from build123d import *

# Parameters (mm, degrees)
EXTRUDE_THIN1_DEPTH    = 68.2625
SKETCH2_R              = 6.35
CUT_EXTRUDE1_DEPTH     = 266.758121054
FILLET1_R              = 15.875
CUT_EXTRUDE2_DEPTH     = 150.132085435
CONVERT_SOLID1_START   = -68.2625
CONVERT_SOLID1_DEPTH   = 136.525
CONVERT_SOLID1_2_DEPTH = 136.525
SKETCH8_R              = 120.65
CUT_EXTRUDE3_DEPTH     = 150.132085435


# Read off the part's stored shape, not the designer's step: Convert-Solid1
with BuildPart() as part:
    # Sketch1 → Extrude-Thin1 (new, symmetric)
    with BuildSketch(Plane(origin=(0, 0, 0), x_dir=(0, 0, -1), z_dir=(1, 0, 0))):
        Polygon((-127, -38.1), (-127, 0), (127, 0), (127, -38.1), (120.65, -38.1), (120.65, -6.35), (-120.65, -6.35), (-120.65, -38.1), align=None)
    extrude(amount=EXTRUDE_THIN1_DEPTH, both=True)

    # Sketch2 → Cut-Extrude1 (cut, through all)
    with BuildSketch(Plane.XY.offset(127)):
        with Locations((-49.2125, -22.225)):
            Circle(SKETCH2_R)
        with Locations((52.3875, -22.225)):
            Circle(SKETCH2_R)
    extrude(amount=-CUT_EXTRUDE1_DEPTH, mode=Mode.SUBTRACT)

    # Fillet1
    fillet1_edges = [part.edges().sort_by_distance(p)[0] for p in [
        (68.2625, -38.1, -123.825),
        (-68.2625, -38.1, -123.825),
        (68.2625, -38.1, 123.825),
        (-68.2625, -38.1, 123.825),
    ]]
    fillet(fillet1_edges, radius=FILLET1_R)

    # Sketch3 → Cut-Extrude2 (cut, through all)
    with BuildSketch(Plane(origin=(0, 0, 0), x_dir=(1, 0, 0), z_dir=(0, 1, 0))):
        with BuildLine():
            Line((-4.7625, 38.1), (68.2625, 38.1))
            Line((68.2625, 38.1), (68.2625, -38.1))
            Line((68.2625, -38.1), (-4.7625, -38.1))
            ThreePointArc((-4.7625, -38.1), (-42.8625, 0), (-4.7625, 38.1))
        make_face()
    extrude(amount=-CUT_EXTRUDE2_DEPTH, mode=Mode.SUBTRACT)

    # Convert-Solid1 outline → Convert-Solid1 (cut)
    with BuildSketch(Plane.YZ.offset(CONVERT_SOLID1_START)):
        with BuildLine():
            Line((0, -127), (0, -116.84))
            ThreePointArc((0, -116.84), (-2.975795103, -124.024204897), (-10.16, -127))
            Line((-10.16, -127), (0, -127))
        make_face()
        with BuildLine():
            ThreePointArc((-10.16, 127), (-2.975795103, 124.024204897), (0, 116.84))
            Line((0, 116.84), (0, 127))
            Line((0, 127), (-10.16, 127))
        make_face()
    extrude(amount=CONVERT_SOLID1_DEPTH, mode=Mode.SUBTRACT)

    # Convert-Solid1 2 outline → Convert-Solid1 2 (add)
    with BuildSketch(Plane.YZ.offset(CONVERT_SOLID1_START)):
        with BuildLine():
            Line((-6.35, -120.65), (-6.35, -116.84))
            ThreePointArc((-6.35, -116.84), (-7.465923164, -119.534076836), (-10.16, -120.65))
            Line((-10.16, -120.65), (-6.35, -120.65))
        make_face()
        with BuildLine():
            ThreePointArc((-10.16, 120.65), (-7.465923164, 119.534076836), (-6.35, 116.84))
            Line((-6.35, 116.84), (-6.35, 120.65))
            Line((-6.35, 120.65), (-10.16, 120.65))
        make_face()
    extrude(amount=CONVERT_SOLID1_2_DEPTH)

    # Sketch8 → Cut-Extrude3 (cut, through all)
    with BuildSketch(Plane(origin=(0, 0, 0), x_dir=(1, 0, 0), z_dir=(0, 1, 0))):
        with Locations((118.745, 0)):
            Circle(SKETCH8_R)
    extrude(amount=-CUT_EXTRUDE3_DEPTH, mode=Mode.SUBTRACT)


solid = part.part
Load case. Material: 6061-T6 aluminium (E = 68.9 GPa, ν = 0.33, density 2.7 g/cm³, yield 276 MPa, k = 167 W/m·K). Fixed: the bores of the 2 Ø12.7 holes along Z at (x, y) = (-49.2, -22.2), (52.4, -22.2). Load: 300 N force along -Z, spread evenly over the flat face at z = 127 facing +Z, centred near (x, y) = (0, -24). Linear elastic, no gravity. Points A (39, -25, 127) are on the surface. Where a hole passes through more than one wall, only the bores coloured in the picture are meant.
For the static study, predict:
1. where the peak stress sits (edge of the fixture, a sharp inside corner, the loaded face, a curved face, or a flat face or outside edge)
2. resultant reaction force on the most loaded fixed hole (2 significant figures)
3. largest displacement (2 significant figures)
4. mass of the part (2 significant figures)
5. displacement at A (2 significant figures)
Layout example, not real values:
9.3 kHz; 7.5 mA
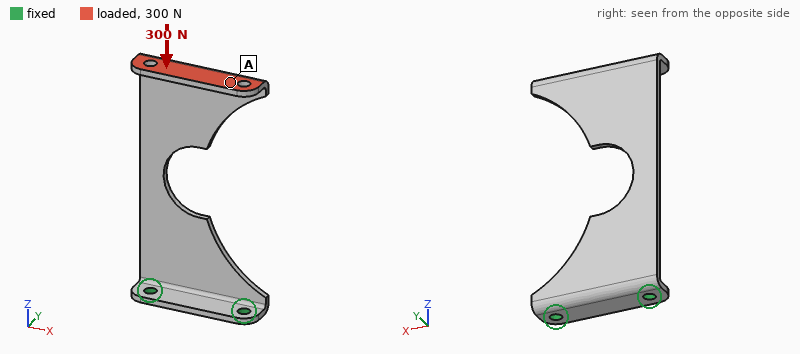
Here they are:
a curved face; 170 N; 2.8 mm; 480 g; 2.7 mm
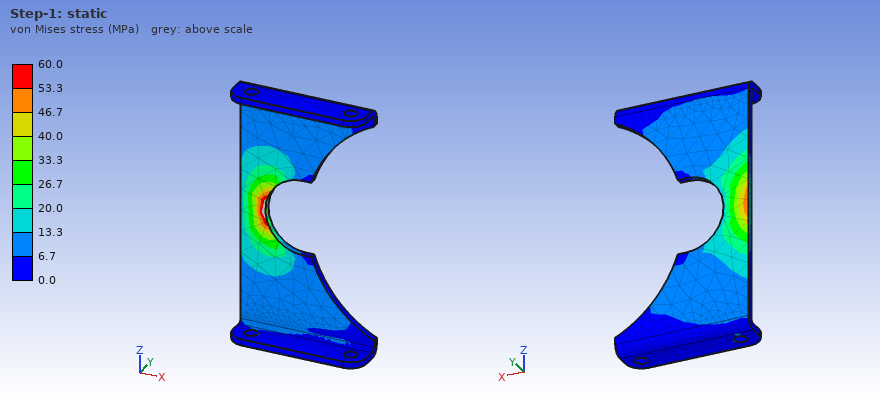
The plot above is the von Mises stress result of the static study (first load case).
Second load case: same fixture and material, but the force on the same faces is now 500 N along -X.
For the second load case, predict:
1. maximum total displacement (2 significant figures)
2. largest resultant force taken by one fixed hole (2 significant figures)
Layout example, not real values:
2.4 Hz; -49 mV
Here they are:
3.2 mm; 1.4 kN
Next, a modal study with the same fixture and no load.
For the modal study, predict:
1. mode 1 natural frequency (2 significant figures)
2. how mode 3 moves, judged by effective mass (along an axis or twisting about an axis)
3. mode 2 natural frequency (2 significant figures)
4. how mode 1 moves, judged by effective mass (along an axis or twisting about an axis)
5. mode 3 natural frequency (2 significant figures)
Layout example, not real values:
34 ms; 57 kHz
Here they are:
47 Hz; along X; 190 Hz; along Y; 280 Hz
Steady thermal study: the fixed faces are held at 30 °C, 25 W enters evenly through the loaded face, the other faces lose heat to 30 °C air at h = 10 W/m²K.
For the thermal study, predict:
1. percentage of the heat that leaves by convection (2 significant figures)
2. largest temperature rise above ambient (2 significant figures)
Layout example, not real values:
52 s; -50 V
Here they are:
63 %; 61 K
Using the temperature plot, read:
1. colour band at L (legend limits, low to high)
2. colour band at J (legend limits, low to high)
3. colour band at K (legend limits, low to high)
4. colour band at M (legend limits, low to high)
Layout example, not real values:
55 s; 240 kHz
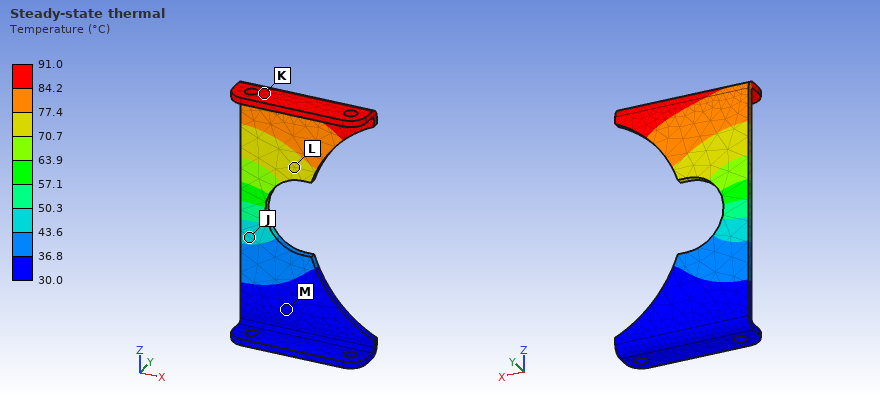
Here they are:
70.7 to 77.4 °C; 43.6 to 50.3 °C; 84.2 to 91.0 °C; 30.0 to 36.8 °C
